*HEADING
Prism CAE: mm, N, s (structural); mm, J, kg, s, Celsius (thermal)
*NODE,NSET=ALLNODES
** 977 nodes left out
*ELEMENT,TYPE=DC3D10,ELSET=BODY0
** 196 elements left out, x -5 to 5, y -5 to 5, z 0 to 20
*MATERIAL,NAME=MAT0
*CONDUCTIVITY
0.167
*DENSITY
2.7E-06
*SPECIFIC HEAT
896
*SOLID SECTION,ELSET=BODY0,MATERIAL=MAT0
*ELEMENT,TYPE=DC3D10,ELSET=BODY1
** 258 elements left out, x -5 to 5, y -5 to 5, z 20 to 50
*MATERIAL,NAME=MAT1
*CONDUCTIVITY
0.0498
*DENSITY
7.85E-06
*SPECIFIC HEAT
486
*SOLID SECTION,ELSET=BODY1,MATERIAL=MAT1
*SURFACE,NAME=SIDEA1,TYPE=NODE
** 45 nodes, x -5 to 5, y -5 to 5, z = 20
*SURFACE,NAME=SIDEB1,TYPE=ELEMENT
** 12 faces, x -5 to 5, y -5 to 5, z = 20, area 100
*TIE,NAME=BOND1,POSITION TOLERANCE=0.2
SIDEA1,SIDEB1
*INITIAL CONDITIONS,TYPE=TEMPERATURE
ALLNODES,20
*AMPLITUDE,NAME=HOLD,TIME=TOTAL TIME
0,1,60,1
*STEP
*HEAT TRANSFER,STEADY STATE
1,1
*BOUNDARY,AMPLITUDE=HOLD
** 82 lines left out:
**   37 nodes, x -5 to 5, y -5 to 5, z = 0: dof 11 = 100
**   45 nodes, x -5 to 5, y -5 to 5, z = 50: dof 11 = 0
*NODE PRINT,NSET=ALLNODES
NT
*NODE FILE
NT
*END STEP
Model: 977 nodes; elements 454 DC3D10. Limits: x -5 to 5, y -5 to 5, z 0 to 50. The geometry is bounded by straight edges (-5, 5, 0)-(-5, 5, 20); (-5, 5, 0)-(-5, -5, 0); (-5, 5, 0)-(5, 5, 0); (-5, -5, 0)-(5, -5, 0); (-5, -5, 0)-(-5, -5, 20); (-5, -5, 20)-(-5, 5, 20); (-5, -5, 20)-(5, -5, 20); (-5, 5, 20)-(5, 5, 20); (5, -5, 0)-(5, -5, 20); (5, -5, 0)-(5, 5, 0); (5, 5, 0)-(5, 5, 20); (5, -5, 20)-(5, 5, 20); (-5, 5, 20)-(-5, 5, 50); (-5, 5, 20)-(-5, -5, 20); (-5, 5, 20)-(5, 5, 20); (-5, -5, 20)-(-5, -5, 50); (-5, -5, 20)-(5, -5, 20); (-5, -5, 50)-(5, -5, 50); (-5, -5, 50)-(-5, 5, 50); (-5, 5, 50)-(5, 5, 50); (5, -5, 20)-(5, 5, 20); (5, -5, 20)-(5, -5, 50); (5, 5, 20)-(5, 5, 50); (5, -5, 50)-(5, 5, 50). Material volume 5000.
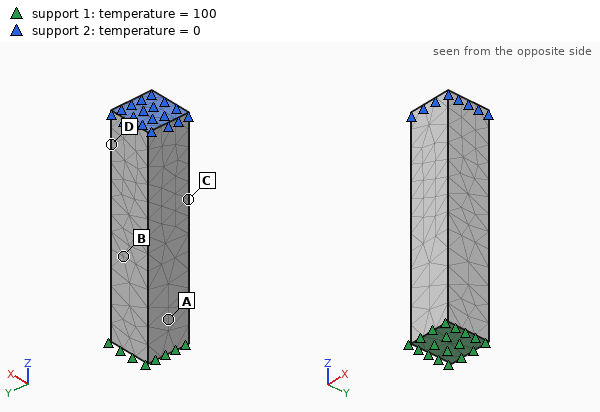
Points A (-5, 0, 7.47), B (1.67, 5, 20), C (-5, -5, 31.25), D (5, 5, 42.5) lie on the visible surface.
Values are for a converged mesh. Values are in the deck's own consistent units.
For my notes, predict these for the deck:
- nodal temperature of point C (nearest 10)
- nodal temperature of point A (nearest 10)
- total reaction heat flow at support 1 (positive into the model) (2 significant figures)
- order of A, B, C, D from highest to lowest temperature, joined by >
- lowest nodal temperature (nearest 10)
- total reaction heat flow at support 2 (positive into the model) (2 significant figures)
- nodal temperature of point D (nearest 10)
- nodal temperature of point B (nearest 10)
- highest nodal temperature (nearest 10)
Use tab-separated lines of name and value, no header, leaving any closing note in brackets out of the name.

nodal temperature of point C	50
nodal temperature of point A	90
total reaction heat flow at support 1 (positive into the model)	14
order of A, B, C, D from highest to lowest temperature, joined by >	A > B > C > D
lowest nodal temperature	0
total reaction heat flow at support 2 (positive into the model)	-14
nodal temperature of point D	20
nodal temperature of point B	80
highest nodal temperature	100
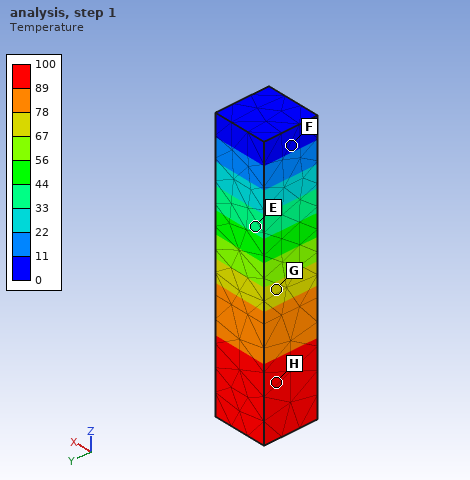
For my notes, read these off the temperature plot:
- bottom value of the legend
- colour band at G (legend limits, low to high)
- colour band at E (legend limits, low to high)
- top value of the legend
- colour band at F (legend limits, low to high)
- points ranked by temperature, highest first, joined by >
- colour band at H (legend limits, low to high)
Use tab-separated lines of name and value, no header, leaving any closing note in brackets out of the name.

bottom value of the legend	0
colour band at G	67 to 78
colour band at E	33 to 44
top value of the legend	100
colour band at F	0 to 11
points ranked by temperature, highest first, joined by >	H > G > E > F
colour band at H	89 to 100
